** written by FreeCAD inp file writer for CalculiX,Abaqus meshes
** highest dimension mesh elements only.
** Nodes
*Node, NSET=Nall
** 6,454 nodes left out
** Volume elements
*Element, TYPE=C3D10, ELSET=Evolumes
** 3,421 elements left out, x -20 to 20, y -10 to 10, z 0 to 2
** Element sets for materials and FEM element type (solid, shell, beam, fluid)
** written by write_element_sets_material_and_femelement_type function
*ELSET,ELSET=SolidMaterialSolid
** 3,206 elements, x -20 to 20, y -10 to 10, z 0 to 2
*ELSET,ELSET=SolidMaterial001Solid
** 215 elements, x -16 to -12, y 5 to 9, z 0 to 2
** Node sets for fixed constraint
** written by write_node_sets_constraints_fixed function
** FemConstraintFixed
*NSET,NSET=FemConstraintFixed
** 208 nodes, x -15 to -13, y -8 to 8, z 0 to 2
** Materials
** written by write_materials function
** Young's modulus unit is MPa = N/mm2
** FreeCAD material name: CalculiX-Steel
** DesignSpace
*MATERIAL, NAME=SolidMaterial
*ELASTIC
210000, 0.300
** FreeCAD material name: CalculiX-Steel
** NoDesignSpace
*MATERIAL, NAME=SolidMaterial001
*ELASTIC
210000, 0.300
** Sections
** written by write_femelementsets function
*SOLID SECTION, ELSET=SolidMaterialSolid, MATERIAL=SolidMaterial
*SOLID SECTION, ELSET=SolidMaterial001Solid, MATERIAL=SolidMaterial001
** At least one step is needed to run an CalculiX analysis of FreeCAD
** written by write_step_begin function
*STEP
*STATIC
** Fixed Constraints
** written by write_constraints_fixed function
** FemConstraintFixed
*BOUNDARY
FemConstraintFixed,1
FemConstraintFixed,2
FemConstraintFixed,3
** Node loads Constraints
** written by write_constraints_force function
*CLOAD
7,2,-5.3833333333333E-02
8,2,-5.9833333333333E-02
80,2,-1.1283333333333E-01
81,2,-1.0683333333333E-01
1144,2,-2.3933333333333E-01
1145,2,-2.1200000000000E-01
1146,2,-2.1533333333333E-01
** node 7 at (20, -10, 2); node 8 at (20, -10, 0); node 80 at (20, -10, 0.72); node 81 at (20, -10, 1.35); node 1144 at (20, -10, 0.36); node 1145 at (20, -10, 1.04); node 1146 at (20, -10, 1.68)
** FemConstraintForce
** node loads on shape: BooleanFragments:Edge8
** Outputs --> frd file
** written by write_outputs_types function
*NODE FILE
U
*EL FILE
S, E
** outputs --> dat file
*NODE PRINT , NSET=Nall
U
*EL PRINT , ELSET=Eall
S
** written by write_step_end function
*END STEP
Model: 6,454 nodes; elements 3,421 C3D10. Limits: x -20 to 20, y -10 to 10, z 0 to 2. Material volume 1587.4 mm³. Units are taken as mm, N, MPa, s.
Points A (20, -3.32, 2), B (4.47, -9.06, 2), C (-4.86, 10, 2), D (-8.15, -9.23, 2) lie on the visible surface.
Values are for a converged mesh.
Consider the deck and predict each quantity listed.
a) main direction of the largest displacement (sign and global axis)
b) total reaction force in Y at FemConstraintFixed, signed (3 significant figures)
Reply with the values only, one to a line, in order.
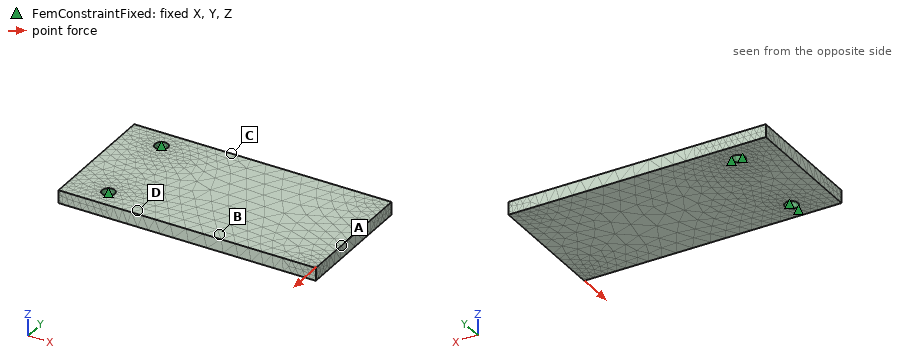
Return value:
-Y
1.00 N
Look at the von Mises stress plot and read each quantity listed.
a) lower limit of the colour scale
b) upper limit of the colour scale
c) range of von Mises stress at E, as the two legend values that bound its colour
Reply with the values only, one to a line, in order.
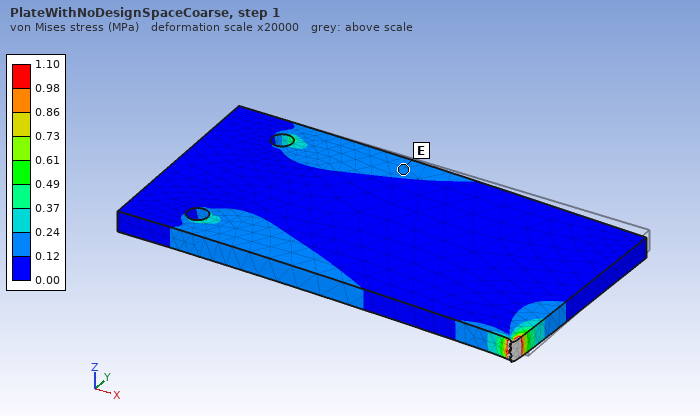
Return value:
0.00 MPa
1.10 MPa
0.12 to 0.24 MPa
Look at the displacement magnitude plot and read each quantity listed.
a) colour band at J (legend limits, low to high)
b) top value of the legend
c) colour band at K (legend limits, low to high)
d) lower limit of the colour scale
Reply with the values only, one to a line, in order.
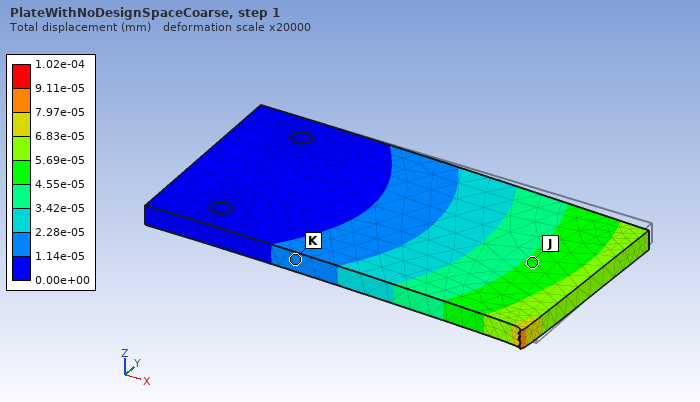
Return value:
4.55e-05 to 5.69e-05 mm
1.02e-04 mm
1.14e-05 to 2.28e-05 mm
0.00e+00 mm
